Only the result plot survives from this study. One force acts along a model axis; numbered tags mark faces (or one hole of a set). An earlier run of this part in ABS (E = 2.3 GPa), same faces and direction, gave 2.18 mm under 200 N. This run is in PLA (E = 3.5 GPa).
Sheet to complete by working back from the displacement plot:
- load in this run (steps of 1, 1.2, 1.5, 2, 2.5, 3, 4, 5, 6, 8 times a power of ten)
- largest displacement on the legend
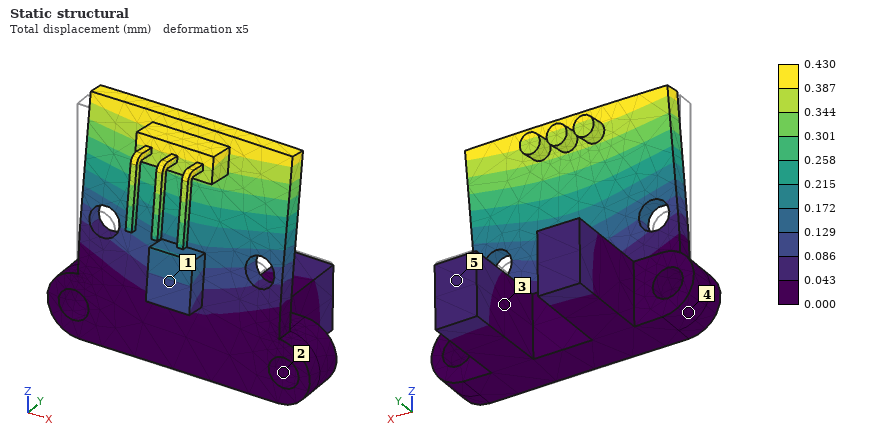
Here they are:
60 N
0.430 mm
